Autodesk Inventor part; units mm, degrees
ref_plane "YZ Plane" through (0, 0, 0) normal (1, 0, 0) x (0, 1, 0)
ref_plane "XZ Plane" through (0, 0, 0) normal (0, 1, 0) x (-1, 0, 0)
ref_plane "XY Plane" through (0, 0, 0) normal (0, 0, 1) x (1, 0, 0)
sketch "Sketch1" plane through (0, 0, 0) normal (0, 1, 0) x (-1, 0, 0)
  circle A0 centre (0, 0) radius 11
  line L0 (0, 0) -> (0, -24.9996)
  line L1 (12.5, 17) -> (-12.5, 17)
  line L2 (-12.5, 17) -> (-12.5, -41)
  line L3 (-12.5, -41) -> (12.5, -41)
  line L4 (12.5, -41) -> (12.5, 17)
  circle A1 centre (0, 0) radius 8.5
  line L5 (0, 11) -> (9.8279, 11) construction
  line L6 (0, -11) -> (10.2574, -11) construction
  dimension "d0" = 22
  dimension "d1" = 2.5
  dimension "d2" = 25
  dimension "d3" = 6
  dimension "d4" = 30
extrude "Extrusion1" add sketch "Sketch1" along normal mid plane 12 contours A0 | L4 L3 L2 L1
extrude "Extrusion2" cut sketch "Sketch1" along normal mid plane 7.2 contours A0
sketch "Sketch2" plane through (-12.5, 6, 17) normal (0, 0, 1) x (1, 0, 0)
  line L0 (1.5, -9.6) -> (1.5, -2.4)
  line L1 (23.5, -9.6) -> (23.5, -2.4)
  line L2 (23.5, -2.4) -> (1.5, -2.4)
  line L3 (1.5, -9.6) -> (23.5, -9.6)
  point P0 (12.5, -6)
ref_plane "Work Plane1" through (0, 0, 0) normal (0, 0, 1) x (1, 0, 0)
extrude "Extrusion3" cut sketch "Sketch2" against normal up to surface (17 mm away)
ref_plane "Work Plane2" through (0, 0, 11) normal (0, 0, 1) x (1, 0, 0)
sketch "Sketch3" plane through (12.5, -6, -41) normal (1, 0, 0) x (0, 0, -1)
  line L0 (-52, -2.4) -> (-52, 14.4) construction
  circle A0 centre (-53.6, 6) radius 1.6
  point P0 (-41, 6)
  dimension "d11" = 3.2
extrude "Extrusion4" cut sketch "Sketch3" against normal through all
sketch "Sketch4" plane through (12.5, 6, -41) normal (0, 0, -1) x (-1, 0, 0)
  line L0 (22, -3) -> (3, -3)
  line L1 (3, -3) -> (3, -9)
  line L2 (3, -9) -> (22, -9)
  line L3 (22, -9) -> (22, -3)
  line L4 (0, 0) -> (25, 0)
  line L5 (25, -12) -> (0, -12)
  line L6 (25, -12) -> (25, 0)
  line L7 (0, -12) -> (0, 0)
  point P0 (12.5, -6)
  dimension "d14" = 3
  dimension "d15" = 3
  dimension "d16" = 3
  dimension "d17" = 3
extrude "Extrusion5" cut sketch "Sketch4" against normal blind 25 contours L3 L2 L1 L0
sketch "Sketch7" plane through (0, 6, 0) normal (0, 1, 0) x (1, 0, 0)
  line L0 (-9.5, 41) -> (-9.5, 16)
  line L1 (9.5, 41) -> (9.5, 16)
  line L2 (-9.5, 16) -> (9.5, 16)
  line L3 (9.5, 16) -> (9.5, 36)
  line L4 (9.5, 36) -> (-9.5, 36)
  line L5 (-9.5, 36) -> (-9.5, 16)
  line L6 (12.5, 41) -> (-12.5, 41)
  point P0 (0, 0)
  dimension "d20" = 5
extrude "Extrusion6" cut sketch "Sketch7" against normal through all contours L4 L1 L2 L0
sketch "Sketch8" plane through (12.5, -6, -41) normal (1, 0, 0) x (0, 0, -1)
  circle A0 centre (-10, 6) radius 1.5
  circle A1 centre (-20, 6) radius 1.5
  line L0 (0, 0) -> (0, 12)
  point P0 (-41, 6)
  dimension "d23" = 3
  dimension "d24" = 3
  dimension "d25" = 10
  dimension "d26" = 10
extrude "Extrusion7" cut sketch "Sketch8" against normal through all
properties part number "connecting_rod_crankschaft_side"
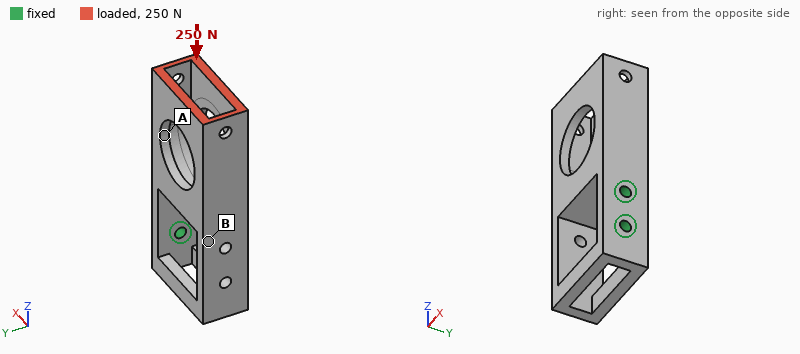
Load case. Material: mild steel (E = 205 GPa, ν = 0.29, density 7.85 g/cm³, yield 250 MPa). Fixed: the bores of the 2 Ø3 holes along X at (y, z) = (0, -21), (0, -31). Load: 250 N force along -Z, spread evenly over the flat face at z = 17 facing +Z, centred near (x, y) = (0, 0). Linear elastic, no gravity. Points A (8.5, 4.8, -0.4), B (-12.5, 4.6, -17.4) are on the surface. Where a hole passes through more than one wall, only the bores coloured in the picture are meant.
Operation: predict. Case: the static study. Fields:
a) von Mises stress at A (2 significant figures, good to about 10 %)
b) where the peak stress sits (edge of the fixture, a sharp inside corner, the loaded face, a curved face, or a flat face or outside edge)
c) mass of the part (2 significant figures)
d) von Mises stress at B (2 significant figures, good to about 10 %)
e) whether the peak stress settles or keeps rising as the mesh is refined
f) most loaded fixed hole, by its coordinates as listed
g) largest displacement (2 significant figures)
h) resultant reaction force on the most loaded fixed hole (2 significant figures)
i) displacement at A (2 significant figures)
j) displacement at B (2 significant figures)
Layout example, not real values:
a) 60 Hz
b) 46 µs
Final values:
a) 9.7 MPa
b) edge of the fixture
c) 55 g
d) 35 MPa
e) keeps rising
f) (0, -21)
g) 42 µm
h) 200 N
i) 18 µm
j) 23 µm
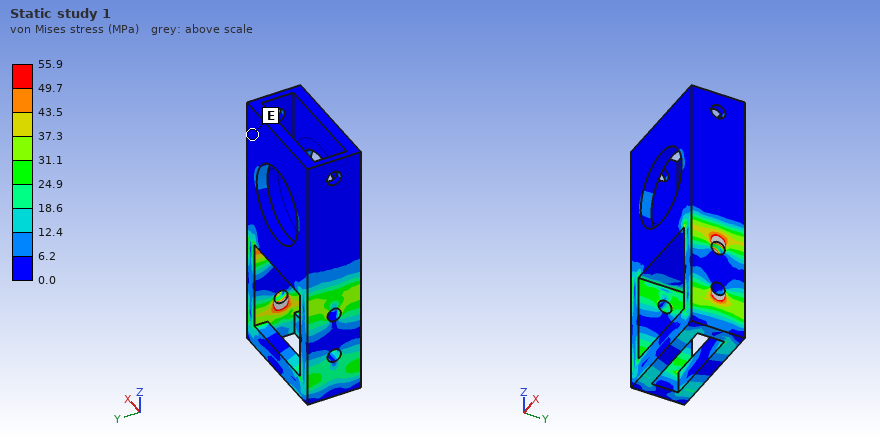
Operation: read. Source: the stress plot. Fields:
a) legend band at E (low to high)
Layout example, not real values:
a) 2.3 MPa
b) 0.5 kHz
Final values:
a) 0.0 to 6.2 MPa
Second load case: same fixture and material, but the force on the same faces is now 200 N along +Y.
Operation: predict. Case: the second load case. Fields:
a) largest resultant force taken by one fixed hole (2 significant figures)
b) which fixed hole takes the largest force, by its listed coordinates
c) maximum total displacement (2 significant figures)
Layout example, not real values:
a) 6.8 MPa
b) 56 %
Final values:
a) 650 N
b) (0, -21)
c) 76 µm
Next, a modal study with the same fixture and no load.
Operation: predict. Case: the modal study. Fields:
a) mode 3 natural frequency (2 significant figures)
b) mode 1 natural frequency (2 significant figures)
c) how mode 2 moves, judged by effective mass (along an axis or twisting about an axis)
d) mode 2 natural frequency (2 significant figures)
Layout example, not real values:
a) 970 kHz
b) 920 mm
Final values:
a) 3600 Hz
b) 1700 Hz
c) along Y
d) 2100 Hz
